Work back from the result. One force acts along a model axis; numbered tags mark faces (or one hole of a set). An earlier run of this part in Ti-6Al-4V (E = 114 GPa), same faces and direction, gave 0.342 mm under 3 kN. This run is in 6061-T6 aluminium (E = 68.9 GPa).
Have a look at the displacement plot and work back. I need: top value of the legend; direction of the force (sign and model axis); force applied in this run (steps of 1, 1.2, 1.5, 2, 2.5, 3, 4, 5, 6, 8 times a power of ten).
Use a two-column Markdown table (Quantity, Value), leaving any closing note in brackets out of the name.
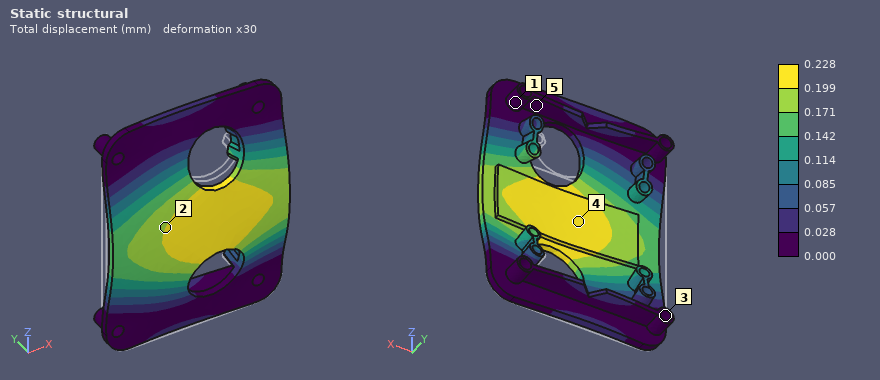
| Quantity | Value |
|---|---|
| top value of the legend | 0.228 mm |
| direction of the force | -Y |
| force applied in this run | 1.2 kN |
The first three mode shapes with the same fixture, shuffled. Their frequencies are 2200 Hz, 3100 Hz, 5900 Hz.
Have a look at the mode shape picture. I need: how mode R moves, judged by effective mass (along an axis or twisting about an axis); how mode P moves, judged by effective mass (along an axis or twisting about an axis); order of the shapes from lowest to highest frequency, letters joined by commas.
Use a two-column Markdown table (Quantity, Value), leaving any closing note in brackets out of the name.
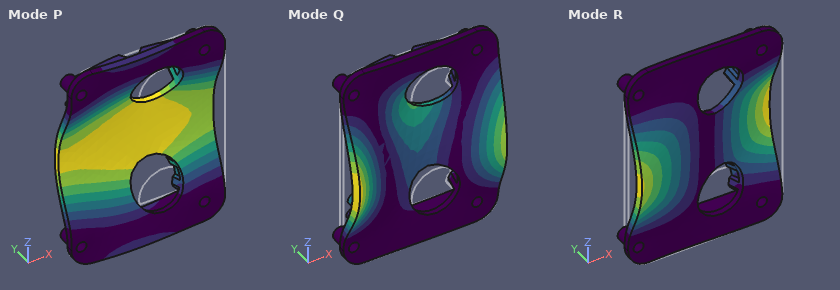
| Quantity | Value |
|---|---|
| how mode R moves, judged by effective mass | twisting about Z |
| how mode P moves, judged by effective mass | along Y |
| order of the shapes from lowest to highest frequency, letters joined by commas | P, R, Q |
